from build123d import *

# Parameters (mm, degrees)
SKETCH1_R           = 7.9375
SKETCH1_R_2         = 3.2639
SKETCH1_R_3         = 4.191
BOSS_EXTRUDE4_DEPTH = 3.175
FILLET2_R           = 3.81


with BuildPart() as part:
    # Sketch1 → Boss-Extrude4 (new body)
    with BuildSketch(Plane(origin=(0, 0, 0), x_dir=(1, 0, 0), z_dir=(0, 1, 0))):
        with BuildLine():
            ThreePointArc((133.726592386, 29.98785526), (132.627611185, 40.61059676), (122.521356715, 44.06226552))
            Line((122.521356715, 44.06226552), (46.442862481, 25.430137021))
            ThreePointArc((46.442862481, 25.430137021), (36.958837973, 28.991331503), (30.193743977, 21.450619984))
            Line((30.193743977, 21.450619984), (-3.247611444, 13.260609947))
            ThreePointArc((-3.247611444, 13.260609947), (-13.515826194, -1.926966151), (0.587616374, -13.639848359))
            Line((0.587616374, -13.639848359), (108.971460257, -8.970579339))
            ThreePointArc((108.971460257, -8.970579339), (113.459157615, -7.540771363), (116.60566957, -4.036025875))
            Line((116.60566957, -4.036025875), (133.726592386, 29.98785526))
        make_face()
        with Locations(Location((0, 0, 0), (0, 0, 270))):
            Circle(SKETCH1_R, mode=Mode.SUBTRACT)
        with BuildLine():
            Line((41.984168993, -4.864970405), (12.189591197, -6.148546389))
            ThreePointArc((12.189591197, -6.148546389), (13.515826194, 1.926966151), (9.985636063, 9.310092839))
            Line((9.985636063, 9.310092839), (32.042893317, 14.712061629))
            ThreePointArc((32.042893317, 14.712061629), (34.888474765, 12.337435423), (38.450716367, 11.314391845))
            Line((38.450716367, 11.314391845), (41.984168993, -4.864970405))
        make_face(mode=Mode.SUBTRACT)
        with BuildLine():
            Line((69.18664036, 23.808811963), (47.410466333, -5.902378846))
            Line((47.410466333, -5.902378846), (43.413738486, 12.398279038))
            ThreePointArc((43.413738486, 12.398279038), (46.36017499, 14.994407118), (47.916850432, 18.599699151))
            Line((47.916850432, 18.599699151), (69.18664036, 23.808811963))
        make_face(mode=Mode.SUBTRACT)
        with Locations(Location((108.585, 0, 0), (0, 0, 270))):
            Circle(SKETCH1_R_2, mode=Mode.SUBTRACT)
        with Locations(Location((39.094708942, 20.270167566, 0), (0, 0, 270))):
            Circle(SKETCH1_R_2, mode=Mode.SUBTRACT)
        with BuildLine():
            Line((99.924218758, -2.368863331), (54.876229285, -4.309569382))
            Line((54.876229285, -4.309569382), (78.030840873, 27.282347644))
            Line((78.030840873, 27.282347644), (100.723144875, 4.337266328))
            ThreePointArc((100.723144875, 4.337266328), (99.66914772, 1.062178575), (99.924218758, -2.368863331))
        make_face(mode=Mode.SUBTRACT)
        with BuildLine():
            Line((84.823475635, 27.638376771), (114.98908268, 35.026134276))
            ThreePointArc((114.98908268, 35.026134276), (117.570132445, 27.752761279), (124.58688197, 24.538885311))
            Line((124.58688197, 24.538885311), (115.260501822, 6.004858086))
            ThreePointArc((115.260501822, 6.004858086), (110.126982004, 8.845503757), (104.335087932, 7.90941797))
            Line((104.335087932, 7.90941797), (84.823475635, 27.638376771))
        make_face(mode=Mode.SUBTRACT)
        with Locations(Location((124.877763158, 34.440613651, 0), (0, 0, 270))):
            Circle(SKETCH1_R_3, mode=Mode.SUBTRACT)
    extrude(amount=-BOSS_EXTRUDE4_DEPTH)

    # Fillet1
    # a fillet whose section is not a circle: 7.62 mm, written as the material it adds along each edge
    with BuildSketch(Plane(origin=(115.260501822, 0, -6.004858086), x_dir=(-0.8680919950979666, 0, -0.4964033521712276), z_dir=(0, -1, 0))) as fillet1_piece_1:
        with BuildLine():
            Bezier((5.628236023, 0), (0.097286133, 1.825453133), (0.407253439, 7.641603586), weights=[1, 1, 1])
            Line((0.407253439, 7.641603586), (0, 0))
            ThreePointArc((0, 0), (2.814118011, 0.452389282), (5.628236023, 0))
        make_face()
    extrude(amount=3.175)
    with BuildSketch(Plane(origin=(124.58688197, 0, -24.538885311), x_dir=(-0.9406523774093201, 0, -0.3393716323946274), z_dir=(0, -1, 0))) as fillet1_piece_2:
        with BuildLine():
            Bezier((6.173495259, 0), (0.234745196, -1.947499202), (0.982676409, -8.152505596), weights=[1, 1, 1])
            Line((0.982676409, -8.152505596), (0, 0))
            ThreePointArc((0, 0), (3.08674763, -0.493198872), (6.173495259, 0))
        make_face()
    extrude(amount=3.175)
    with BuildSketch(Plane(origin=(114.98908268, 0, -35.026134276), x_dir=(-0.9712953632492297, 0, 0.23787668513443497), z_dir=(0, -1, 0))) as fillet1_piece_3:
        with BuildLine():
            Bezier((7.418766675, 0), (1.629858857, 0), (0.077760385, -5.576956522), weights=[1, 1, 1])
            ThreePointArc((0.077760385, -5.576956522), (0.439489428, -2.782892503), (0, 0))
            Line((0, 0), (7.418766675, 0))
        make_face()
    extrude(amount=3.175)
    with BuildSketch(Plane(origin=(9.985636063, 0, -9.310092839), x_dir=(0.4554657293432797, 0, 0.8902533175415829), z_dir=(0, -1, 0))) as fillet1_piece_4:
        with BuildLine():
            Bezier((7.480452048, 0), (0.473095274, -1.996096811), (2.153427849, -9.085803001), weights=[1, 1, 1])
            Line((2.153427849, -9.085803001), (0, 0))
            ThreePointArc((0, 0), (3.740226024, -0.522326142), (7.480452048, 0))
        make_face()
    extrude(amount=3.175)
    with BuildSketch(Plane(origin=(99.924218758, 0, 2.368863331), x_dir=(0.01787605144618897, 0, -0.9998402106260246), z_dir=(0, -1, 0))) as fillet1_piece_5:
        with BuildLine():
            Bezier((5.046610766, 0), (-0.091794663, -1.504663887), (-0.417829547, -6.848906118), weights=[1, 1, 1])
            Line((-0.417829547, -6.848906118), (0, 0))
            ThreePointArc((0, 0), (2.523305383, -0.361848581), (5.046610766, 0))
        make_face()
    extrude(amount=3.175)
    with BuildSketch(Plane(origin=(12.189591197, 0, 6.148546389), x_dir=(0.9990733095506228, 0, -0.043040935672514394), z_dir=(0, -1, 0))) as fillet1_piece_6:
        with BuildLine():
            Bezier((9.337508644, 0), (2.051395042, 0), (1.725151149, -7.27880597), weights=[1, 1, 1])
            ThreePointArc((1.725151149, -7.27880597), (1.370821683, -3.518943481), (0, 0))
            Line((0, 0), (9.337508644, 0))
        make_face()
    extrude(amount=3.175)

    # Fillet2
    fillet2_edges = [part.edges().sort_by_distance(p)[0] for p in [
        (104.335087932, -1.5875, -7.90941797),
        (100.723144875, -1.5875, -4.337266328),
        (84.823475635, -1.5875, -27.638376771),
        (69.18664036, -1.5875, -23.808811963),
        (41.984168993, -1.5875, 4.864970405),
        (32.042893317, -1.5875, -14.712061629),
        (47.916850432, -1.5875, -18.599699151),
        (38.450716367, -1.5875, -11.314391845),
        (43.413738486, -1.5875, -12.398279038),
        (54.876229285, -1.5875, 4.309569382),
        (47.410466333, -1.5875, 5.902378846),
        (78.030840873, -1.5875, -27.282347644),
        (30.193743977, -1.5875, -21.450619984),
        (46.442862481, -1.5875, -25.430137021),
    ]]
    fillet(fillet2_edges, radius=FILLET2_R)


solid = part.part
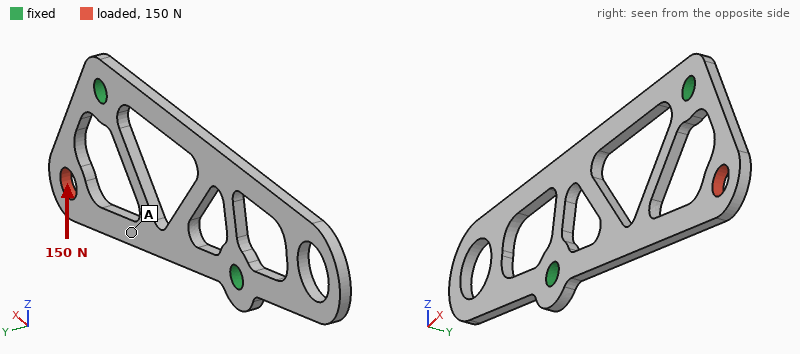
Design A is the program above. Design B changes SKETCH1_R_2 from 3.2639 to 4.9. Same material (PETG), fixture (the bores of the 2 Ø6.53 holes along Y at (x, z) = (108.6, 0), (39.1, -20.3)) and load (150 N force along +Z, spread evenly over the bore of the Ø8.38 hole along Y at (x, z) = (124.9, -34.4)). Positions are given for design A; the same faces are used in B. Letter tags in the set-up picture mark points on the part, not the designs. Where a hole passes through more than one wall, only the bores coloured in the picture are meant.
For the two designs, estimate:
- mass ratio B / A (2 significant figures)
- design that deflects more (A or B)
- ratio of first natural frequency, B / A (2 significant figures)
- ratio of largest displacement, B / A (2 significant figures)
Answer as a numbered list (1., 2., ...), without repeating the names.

1. 0.97
2. A
3. 1.0
4. 0.91
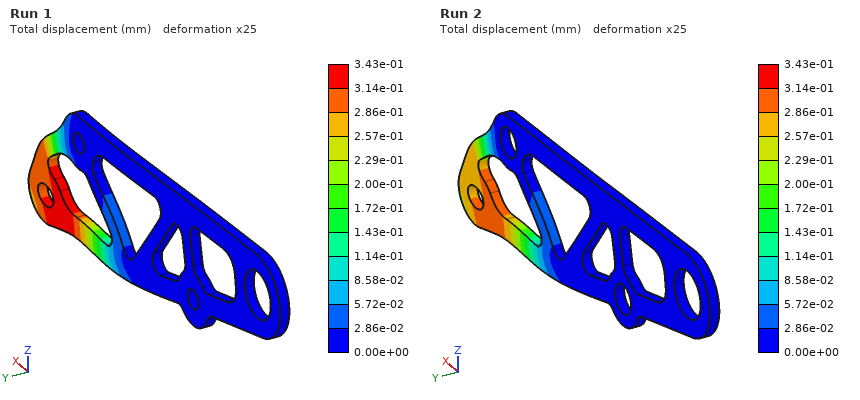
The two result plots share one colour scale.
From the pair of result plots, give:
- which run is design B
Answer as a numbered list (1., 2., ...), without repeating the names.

1. Run 2
